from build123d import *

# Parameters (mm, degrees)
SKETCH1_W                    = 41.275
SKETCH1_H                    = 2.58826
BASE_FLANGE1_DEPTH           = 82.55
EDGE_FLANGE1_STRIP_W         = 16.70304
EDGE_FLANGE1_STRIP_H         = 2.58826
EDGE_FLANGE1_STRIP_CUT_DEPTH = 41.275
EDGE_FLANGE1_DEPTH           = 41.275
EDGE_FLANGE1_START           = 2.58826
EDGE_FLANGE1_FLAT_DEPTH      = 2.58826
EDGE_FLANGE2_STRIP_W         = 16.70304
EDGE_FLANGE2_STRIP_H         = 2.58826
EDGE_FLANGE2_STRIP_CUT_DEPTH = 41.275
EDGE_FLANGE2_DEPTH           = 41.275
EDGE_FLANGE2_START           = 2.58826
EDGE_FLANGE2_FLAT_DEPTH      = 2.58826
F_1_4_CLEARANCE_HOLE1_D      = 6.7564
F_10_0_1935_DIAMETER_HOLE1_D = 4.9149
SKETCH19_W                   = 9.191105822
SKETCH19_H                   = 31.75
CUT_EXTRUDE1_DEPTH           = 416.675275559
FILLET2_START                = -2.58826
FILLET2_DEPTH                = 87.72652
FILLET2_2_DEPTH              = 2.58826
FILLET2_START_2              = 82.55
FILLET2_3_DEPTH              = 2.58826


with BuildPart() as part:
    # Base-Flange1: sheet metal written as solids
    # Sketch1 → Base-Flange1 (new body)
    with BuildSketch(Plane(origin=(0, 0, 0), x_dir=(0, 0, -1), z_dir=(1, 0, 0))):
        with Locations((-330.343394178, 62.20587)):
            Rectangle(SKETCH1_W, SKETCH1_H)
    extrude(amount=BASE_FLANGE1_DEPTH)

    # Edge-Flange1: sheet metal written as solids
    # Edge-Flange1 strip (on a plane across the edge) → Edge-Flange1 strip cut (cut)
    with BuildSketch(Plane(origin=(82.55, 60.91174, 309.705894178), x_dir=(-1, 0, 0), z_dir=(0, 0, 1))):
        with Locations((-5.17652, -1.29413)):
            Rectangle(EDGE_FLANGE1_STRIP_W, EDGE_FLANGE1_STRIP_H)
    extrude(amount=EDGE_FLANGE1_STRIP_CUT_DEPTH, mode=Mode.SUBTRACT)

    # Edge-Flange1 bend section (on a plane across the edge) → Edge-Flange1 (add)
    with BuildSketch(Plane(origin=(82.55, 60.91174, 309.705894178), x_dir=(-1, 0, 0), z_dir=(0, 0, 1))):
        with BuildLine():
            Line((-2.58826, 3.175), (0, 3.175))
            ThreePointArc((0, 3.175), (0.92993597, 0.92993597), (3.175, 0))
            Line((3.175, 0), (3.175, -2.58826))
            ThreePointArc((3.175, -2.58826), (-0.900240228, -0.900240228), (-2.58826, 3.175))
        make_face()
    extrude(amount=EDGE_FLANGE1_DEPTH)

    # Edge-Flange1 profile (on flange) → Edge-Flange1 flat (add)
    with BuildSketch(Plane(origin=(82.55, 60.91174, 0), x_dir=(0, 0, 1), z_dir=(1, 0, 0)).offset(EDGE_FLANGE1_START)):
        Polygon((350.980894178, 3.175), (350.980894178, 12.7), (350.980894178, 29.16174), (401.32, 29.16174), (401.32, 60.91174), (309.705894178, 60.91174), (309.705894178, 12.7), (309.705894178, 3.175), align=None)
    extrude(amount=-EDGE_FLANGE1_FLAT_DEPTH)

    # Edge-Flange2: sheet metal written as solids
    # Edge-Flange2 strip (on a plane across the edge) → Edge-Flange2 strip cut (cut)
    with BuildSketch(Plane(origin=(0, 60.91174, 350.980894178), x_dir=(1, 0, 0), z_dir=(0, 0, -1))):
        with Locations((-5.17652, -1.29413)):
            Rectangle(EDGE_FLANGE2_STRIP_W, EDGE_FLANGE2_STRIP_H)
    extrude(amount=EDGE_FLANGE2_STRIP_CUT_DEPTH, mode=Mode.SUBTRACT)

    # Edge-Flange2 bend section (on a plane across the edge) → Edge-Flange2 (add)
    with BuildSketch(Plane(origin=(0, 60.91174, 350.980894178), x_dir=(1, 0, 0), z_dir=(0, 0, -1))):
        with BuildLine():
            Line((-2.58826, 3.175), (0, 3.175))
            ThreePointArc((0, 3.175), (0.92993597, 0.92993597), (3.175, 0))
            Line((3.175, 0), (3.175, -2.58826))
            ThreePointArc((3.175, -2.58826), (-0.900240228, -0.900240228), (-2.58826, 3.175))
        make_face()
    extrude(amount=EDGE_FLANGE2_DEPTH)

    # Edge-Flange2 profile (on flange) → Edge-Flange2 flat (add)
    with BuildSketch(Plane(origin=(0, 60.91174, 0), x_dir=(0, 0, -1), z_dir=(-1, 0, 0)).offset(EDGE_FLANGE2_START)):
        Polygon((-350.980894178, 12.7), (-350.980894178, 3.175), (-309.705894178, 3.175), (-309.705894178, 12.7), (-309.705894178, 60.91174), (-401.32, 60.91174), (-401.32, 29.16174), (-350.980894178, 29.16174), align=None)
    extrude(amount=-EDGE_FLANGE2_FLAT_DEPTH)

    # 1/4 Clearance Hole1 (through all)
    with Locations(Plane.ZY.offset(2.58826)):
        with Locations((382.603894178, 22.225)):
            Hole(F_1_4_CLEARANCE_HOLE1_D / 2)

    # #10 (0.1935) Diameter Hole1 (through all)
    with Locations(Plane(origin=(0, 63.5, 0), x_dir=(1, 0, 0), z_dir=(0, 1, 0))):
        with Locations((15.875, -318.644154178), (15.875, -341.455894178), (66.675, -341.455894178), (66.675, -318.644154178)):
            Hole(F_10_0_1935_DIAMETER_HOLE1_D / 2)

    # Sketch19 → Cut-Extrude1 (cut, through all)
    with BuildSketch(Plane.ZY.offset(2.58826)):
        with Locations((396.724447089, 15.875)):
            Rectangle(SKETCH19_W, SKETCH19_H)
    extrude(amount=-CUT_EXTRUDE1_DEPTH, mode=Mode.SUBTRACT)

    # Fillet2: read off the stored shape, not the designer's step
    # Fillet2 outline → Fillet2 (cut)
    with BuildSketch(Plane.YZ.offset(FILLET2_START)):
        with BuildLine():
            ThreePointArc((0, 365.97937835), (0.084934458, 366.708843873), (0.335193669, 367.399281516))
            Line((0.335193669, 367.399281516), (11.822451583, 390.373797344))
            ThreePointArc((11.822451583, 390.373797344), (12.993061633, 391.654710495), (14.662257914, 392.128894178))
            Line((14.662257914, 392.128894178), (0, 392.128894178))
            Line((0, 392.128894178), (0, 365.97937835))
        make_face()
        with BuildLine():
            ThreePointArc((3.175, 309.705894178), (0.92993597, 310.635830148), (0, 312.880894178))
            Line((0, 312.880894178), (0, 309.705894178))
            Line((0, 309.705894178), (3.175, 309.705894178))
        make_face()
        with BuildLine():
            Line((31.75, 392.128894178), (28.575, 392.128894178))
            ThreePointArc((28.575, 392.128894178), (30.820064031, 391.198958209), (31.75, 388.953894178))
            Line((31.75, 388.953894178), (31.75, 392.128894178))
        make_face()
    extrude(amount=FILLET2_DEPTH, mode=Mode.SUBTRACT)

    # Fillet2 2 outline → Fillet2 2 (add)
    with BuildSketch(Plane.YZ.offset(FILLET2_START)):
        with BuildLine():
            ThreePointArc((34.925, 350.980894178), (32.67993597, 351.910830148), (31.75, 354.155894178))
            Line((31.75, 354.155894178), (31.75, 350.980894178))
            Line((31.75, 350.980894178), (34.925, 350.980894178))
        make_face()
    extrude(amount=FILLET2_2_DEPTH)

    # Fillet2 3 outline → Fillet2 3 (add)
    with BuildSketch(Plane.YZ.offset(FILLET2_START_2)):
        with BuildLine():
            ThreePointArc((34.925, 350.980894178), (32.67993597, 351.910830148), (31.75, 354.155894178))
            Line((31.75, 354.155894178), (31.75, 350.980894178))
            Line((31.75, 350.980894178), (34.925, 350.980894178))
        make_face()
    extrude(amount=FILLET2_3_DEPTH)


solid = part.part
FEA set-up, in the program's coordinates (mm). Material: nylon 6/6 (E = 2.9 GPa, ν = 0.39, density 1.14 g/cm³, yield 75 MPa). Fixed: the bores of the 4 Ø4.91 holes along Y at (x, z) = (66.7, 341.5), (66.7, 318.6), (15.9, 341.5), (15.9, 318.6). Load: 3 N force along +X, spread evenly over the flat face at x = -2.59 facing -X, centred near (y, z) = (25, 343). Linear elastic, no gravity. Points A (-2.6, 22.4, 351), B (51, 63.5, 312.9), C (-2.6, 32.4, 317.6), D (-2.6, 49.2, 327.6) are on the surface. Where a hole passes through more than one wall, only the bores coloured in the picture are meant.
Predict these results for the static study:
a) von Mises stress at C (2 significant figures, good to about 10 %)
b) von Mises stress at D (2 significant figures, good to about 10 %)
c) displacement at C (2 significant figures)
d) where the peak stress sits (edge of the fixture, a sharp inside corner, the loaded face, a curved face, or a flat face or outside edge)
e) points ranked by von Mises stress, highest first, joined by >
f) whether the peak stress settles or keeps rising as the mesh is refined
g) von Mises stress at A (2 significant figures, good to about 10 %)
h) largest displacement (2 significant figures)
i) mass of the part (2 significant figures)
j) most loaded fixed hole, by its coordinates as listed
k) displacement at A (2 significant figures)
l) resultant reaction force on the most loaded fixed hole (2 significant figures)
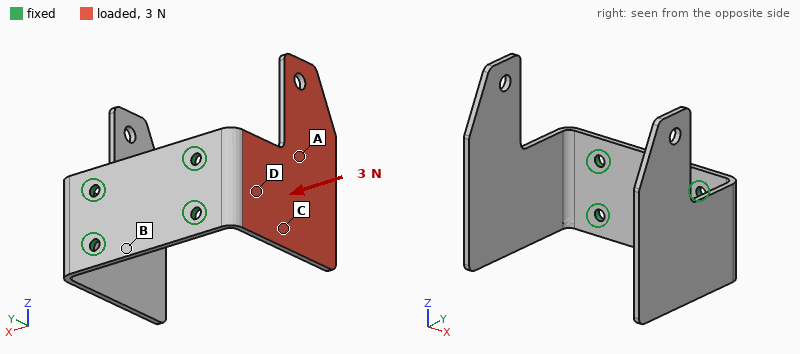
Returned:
0.83 MPa
1.5 MPa
0.40 mm
edge of the fixture
D > C > A > B
keeps rising
0.55 MPa
1.3 mm
31 g
(15.9, 341.5)
0.74 mm
2.9 N
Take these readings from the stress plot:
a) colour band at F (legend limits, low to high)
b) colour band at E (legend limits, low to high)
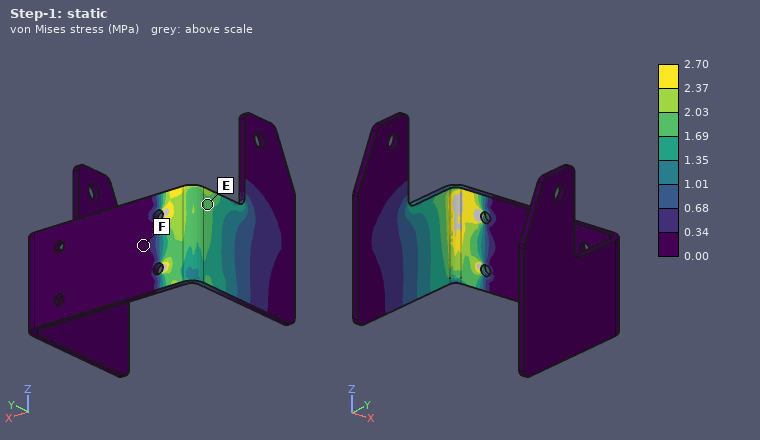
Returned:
0.00 to 0.34 MPa
1.69 to 2.03 MPa
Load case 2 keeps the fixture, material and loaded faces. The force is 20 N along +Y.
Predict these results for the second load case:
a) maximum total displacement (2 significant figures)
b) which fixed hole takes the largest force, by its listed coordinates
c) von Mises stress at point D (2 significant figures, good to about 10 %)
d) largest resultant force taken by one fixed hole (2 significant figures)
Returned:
1.5 mm
(15.9, 341.5)
0.90 MPa
20 N
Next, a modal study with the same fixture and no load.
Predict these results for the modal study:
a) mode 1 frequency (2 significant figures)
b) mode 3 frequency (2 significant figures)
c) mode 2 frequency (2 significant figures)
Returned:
92 Hz
190 Hz
92 Hz
